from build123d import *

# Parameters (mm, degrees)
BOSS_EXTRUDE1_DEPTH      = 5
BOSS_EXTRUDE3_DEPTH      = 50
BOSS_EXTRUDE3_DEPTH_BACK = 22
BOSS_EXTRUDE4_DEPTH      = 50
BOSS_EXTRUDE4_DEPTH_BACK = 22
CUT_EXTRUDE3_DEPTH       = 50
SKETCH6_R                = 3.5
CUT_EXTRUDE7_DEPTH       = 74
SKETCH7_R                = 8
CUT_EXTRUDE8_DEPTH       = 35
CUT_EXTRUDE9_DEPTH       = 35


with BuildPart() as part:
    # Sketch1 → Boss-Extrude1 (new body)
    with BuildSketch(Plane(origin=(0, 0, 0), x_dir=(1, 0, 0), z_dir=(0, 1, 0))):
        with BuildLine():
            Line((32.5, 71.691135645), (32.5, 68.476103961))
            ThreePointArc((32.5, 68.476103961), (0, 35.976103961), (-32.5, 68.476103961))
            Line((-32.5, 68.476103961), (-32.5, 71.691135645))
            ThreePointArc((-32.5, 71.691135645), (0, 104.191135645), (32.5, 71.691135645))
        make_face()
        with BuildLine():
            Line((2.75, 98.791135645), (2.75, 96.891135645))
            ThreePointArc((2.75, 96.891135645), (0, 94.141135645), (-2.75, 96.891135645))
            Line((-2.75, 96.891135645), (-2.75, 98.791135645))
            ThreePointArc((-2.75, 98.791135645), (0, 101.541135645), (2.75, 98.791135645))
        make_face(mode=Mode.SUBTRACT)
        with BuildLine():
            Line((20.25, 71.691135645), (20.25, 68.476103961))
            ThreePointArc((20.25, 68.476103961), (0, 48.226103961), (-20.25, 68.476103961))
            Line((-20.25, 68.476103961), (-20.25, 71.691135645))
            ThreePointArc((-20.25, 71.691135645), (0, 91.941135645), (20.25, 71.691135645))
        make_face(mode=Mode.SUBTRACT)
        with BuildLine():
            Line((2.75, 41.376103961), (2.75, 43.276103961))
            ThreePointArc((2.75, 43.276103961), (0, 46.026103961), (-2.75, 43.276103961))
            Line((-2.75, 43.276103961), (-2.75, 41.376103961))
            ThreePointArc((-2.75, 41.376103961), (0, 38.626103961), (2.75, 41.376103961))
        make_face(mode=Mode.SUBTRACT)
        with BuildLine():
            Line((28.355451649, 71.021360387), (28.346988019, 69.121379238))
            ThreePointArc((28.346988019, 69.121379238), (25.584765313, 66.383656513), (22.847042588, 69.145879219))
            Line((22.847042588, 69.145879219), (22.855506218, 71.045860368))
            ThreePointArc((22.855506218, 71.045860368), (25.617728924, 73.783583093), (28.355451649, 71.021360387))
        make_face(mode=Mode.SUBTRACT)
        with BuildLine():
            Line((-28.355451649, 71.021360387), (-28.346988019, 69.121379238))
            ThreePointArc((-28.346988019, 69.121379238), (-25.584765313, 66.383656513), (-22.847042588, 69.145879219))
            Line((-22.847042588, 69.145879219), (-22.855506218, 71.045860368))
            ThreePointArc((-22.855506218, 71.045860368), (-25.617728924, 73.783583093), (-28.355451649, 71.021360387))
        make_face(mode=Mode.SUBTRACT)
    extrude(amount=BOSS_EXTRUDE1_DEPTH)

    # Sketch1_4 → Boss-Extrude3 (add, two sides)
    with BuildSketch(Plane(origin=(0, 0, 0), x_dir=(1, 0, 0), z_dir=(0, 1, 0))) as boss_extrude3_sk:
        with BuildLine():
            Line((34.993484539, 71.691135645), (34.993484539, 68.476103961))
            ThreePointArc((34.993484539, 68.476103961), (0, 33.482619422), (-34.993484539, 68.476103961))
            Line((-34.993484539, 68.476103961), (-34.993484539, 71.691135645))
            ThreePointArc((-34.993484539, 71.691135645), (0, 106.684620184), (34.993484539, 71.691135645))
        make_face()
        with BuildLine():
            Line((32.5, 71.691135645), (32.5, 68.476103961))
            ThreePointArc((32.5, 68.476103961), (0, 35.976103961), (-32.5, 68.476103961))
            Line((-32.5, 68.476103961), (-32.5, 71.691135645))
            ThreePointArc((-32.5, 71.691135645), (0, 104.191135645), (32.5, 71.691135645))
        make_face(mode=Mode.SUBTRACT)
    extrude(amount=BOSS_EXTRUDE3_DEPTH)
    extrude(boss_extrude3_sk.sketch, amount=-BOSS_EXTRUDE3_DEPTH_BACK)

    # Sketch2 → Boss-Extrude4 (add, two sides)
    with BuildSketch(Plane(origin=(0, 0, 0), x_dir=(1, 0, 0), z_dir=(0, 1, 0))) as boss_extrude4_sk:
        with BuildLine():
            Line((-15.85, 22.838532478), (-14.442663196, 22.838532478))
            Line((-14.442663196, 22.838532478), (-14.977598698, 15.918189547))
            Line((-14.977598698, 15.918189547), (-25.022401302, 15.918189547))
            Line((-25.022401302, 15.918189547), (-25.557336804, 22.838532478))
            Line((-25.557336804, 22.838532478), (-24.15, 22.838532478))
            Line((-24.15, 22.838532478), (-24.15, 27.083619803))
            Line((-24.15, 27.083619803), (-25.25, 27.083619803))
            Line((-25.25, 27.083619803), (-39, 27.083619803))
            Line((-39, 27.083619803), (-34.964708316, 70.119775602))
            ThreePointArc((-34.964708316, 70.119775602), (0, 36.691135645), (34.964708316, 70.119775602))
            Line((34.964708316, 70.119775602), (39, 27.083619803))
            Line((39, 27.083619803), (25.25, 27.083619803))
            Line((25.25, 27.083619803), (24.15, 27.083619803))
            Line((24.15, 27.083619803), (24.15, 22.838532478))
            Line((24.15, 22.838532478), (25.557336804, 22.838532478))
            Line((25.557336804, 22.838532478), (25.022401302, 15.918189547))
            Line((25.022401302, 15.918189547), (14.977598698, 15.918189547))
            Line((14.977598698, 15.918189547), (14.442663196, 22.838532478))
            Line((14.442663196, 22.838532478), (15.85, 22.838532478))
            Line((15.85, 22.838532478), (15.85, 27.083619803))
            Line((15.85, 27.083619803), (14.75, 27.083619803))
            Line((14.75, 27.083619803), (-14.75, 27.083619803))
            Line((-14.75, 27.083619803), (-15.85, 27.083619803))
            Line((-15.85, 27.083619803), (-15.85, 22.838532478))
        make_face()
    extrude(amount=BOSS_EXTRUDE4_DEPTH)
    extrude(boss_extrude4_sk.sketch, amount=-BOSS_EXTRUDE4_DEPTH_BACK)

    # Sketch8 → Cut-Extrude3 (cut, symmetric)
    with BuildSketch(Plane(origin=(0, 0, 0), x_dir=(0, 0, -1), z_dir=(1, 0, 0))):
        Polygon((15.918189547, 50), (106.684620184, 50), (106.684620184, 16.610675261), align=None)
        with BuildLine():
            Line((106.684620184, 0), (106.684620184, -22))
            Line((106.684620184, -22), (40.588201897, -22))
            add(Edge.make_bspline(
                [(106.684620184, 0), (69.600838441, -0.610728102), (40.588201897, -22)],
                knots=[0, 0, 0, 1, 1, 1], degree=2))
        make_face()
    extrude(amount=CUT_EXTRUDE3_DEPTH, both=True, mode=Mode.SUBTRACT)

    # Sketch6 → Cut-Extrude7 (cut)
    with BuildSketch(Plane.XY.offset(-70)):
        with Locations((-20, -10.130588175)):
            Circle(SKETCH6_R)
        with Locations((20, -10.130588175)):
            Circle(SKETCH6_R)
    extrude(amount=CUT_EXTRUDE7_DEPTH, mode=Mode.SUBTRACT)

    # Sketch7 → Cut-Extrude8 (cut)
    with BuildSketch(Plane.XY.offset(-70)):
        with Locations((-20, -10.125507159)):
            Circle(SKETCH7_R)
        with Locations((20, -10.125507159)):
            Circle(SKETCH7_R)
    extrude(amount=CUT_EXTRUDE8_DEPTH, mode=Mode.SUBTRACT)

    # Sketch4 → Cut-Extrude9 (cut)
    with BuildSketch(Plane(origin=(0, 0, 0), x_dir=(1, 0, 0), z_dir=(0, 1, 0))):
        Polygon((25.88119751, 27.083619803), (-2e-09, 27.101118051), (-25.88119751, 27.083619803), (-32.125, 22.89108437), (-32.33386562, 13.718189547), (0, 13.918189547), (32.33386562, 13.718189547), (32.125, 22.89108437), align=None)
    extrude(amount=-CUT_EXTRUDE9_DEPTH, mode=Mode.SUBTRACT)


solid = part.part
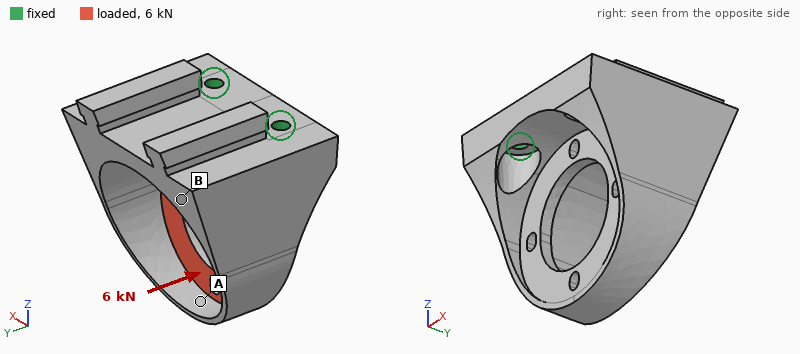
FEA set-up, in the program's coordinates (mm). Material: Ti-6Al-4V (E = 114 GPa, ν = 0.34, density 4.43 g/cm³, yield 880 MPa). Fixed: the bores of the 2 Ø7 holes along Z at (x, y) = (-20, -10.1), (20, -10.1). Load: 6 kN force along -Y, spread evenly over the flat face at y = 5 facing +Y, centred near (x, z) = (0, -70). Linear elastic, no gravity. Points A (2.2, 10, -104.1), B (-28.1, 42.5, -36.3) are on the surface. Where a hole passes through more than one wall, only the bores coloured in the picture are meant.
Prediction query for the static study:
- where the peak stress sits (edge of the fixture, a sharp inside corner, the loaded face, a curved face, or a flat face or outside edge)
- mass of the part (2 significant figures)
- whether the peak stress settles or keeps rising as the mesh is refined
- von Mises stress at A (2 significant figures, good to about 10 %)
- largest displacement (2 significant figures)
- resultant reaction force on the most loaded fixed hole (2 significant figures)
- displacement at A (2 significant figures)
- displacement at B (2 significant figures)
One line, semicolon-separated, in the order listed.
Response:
edge of the fixture; 490 g; keeps rising; 89 MPa; 0.47 mm; 3.0 kN; 0.42 mm; 0.19 mm
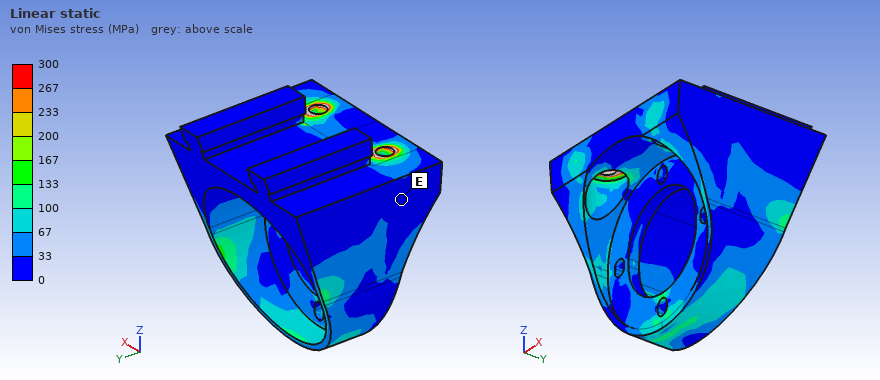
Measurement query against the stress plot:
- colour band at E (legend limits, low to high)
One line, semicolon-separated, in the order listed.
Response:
0 to 33 MPa
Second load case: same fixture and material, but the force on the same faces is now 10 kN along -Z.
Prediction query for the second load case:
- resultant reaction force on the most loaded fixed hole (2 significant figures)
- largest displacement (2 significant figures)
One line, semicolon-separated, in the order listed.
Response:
5.0 kN; 0.20 mm
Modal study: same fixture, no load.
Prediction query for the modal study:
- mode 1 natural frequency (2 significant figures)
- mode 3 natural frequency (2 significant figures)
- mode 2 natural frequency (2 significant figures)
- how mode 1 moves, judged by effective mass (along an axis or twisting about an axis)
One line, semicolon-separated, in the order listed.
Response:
1600 Hz; 4300 Hz; 3000 Hz; along Z
